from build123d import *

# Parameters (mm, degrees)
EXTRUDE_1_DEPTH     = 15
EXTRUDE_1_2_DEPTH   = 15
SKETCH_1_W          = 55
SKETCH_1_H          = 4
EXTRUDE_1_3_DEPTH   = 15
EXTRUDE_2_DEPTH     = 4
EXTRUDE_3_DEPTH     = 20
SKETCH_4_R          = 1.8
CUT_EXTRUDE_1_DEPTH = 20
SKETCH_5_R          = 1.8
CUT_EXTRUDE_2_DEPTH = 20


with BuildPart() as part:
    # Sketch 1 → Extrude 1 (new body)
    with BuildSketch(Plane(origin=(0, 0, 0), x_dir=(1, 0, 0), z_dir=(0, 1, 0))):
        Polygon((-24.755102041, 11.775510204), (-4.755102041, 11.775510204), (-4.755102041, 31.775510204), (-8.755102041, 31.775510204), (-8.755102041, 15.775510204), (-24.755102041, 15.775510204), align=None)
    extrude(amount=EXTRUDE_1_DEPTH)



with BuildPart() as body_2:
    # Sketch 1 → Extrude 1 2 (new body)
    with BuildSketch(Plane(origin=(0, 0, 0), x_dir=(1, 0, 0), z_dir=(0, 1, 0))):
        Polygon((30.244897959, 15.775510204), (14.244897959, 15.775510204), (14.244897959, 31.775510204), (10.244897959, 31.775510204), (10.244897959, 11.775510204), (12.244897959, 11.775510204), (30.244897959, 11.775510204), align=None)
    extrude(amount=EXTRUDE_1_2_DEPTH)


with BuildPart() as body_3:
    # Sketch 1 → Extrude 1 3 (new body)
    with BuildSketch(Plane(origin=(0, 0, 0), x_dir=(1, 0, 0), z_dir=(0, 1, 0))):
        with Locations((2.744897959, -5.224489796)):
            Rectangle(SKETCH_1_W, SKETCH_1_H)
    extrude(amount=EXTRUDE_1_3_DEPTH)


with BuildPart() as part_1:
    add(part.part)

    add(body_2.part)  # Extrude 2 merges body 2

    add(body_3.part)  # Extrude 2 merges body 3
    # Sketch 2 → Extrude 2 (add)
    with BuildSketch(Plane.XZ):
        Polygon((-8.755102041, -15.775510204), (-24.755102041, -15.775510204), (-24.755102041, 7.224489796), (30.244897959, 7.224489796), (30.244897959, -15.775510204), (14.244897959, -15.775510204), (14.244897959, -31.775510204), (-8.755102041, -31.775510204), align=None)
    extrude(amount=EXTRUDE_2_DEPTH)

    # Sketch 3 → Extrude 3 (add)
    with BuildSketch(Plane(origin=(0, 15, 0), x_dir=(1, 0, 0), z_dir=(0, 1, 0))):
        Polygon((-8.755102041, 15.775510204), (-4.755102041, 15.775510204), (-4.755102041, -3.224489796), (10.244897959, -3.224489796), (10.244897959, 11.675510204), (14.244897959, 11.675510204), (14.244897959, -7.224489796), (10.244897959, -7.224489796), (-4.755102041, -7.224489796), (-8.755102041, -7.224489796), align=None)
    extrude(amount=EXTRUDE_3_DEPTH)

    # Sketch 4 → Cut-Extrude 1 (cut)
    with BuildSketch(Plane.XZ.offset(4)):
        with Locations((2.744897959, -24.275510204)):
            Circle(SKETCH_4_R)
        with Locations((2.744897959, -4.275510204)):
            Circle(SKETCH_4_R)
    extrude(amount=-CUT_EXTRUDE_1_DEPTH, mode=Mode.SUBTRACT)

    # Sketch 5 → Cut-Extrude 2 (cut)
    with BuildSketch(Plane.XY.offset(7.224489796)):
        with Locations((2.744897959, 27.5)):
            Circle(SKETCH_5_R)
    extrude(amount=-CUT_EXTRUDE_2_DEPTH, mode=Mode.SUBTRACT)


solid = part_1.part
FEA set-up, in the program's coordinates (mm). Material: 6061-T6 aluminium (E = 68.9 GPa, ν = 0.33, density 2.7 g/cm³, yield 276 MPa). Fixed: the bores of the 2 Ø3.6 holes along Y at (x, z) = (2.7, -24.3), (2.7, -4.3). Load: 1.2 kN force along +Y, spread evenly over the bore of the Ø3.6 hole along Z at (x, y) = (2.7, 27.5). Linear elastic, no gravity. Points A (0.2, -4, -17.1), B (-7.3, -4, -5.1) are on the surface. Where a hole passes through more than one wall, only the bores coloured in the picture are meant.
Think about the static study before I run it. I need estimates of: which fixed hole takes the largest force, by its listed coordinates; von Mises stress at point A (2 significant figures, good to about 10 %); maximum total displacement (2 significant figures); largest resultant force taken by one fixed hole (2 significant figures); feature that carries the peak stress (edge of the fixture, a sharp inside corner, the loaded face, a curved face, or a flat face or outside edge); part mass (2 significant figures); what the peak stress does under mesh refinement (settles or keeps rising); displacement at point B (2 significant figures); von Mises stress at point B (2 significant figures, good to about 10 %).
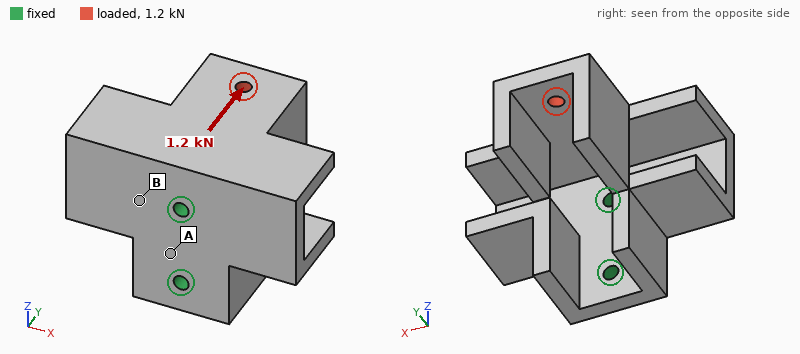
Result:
(2.7, -4.3)
12 MPa
75 µm
1.5 kN
edge of the fixture
50 g
keeps rising
11 µm
29 MPa
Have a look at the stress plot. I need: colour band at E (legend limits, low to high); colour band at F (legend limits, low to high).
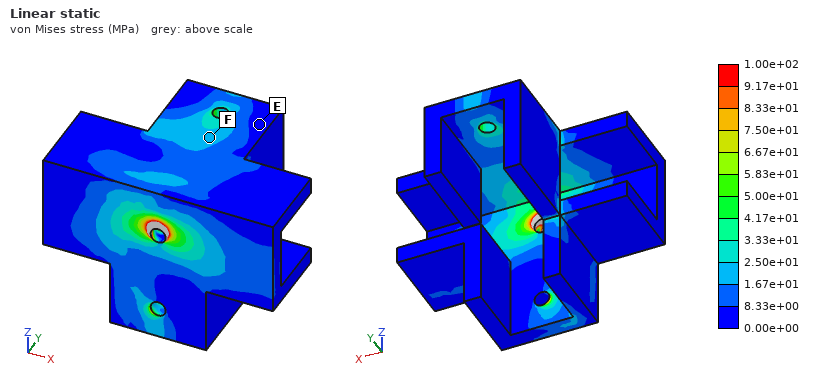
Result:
0.00e+00 to 8.33e+00 MPa
1.67e+01 to 2.50e+01 MPa
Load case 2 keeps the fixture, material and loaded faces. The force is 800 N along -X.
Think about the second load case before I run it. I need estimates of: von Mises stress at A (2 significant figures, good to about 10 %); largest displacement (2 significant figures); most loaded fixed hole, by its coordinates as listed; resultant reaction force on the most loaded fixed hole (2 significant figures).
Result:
56 MPa
0.41 mm
(2.7, -4.3)
1.1 kN
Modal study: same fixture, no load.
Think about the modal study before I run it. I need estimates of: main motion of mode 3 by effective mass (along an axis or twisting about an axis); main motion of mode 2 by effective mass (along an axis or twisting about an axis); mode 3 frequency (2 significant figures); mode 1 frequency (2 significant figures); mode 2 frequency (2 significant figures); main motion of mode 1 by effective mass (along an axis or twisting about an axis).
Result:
along Y
along Z
5000 Hz
1900 Hz
3100 Hz
along X
